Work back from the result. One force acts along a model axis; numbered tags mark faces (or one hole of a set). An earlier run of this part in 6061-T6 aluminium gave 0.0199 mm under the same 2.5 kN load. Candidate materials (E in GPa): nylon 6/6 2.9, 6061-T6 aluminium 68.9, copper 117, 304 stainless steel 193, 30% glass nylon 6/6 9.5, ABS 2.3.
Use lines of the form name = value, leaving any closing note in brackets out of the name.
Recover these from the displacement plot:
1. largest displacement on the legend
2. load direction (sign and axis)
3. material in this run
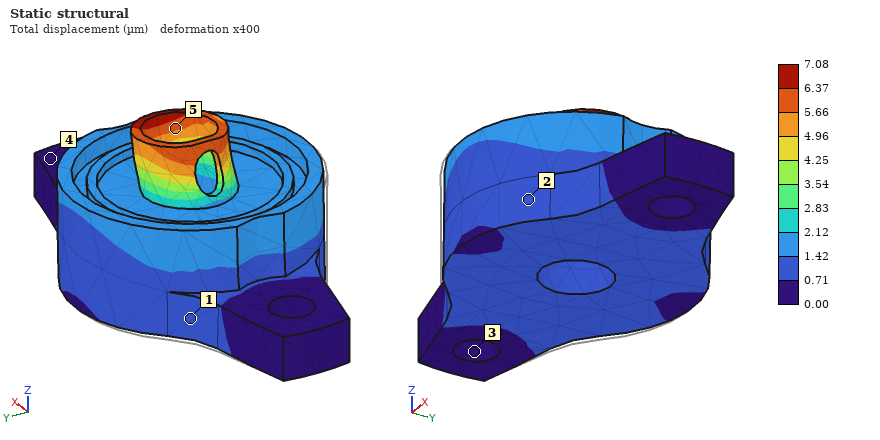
largest displacement on the legend = 7.08 µm
load direction = +X
material in this run = 304 stainless steel
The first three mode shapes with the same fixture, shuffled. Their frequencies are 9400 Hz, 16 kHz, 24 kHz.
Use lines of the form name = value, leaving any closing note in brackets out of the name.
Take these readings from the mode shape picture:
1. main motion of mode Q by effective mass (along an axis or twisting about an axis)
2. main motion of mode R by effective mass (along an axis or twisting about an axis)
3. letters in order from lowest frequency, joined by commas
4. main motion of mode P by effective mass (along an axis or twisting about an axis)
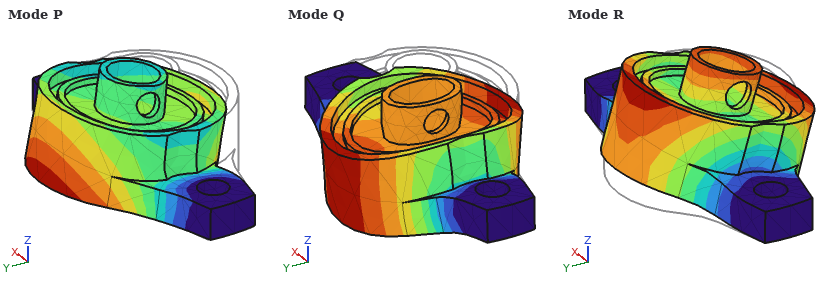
main motion of mode Q by effective mass = along Z
main motion of mode R by effective mass = along Y
letters in order from lowest frequency, joined by commas = R, Q, P
main motion of mode P by effective mass = along Y
